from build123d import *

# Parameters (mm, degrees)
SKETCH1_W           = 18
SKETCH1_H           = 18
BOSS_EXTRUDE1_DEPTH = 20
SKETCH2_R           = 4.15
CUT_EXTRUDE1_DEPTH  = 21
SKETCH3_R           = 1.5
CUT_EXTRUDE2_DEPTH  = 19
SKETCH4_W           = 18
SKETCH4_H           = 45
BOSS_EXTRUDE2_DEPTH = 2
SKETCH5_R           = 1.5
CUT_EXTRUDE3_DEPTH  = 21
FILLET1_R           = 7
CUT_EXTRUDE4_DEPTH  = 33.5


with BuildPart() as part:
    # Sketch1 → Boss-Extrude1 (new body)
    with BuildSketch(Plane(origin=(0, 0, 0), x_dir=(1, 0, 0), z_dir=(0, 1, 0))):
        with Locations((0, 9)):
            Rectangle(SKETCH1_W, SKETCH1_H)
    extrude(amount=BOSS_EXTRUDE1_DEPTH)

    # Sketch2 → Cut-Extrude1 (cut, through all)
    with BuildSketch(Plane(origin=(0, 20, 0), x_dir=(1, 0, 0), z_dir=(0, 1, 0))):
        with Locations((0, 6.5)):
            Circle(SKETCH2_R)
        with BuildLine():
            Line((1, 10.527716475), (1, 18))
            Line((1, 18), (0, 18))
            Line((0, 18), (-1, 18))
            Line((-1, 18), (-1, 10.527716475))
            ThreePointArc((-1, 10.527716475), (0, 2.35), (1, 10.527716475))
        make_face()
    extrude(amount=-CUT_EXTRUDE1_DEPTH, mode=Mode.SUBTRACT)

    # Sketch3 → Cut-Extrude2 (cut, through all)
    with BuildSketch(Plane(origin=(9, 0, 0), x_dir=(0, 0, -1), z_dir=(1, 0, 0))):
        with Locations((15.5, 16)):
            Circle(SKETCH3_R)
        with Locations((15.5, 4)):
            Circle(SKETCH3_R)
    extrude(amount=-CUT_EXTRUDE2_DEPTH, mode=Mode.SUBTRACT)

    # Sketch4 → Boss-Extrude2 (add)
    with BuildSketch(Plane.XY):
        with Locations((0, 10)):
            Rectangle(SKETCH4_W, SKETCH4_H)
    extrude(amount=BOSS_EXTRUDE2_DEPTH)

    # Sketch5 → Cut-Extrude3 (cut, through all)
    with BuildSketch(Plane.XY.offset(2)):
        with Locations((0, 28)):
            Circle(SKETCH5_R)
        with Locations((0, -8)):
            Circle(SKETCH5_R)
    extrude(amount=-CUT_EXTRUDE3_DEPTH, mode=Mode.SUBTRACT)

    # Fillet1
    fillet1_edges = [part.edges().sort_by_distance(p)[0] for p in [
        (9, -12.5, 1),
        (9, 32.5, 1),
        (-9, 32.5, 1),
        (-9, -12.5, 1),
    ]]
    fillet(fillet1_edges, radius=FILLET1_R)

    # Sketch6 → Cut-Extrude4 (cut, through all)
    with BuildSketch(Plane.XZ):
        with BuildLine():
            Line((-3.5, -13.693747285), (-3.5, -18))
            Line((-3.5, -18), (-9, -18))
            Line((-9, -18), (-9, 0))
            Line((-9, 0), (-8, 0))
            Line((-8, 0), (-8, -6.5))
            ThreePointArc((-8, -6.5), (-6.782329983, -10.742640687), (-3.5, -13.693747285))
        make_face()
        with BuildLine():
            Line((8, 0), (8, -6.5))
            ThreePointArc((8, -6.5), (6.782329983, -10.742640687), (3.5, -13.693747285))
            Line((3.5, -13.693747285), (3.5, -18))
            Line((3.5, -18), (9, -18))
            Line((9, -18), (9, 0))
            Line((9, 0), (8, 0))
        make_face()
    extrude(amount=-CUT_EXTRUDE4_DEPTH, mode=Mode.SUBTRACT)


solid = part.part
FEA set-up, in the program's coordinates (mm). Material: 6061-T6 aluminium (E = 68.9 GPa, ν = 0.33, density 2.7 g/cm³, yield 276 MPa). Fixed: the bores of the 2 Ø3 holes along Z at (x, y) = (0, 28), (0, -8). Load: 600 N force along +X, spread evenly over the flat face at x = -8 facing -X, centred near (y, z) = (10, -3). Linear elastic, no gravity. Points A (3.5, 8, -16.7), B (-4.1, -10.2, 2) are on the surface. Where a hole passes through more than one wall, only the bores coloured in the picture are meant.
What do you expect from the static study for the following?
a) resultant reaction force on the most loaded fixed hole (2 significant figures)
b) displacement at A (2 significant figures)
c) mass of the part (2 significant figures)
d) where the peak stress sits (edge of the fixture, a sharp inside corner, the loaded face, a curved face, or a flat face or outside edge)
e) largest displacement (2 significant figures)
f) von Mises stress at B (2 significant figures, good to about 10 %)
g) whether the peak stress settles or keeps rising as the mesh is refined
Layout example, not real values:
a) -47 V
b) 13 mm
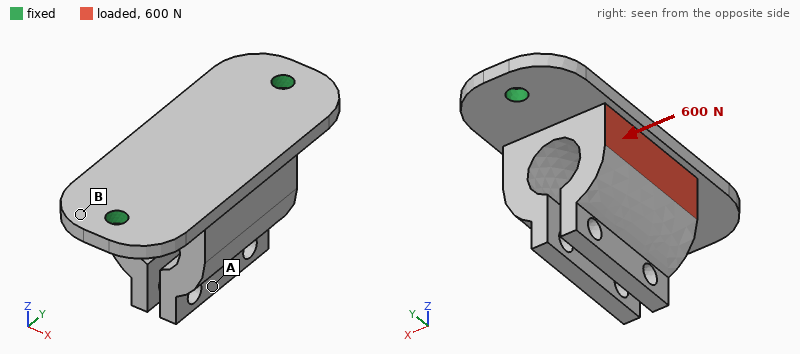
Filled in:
a) 300 N
b) 0.13 mm
c) 13 g
d) edge of the fixture
e) 0.15 mm
f) 60 MPa
g) keeps rising
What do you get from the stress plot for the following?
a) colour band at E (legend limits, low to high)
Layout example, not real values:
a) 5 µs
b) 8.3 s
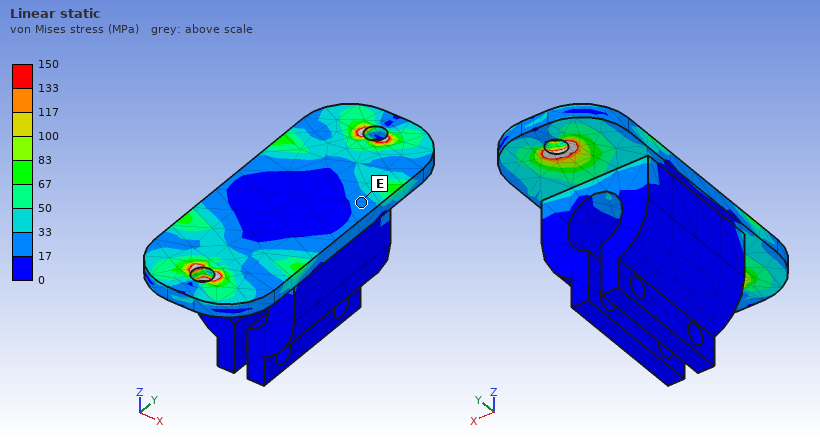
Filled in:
a) 17 to 33 MPa
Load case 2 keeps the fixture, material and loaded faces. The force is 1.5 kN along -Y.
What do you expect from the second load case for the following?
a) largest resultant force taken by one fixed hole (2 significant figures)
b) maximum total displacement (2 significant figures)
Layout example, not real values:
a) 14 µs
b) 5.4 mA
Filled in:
a) 850 N
b) 41 µm
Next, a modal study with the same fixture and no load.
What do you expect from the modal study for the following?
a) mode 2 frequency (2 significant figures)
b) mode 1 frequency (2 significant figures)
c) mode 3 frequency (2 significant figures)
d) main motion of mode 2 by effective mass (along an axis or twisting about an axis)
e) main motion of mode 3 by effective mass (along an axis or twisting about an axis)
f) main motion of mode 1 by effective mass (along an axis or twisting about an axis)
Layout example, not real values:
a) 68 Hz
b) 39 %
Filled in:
a) 6600 Hz
b) 2900 Hz
c) 8700 Hz
d) along Z
e) along Y
f) along X
